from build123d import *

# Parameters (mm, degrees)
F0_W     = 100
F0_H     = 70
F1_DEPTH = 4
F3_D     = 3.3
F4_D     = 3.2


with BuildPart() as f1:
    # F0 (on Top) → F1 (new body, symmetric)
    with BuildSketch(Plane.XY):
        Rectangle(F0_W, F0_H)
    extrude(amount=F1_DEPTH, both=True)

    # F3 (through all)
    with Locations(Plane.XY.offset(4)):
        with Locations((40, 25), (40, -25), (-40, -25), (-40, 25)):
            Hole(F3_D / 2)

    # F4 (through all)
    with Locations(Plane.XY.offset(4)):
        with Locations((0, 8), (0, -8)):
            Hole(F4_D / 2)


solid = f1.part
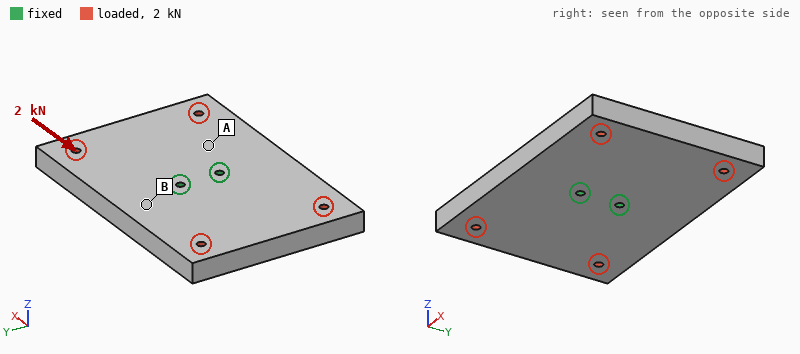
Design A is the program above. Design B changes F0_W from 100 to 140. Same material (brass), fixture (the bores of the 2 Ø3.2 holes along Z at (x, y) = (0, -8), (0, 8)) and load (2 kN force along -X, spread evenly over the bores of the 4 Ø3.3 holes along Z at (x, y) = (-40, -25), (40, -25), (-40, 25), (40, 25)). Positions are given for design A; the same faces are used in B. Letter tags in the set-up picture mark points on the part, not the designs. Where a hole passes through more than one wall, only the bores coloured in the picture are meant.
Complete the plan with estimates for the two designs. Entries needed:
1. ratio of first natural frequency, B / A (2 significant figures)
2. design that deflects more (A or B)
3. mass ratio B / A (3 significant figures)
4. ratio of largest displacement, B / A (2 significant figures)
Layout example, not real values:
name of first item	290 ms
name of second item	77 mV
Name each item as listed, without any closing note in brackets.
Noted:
ratio of first natural frequency, B / A	0.56
design that deflects more	A
mass ratio B / A	1.40
ratio of largest displacement, B / A	0.90
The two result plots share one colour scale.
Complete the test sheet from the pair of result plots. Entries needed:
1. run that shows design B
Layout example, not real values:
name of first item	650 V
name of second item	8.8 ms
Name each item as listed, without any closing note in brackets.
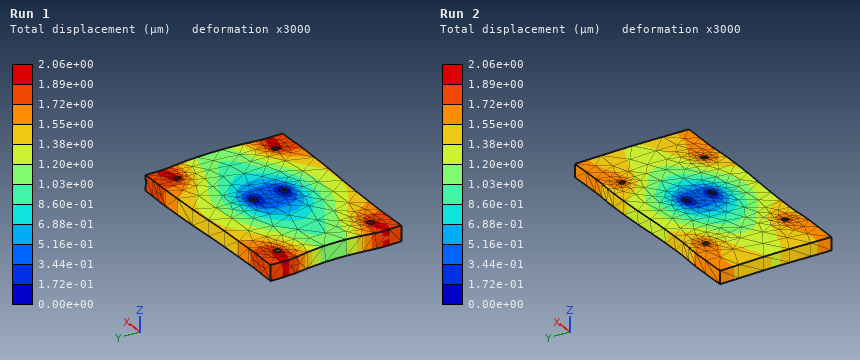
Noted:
run that shows design B	Run 2
